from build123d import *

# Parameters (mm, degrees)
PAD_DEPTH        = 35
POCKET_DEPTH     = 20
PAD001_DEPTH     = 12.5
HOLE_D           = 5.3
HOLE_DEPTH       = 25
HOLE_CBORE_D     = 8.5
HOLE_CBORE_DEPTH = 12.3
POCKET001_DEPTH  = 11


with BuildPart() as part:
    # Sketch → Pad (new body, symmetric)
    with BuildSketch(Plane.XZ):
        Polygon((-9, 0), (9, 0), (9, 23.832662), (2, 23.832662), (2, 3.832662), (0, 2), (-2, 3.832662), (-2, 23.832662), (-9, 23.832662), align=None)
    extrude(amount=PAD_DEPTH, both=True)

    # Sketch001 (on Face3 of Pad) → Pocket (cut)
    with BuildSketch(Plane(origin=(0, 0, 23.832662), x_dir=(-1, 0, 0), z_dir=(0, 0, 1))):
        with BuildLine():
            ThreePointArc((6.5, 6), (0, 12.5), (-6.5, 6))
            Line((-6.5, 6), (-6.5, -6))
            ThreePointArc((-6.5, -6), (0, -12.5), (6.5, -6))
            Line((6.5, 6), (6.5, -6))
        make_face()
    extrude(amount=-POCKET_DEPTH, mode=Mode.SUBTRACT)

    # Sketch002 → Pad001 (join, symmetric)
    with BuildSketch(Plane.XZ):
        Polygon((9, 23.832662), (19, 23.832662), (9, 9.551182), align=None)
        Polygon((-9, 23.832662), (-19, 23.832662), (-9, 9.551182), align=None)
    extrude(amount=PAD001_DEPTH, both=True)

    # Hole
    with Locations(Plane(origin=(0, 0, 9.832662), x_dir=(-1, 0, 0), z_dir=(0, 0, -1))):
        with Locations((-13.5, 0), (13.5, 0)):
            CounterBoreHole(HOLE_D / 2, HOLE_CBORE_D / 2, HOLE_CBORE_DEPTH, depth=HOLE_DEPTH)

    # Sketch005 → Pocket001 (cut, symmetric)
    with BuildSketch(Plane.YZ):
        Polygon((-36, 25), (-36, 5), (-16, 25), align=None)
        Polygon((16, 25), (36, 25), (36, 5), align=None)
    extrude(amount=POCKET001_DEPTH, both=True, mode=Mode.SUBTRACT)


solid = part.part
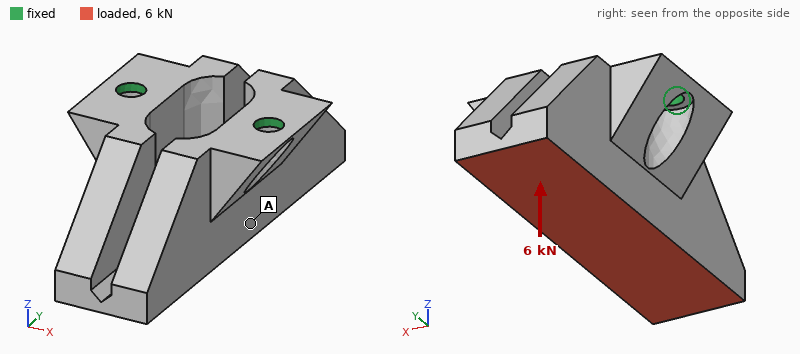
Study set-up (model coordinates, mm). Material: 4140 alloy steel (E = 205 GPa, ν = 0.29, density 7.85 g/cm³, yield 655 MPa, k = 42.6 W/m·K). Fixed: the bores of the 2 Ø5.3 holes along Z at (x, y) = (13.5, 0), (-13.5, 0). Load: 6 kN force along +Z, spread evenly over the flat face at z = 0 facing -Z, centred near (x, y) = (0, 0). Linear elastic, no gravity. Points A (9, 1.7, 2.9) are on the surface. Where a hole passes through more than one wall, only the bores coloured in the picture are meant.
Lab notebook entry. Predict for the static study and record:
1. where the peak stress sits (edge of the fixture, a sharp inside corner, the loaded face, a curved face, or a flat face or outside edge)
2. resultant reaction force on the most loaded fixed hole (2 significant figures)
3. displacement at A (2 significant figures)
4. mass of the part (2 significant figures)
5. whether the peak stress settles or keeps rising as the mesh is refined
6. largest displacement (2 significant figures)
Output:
edge of the fixture
3.2 kN
8.5 µm
150 g
keeps rising
16 µm
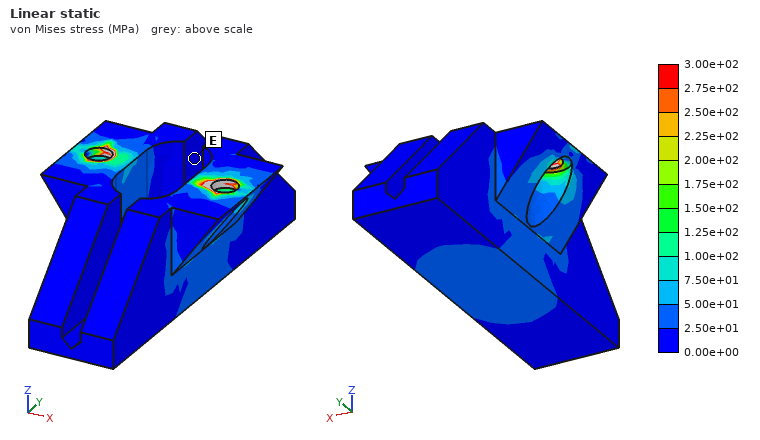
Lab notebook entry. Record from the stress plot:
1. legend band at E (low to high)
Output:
0.00e+00 to 2.50e+01 MPa
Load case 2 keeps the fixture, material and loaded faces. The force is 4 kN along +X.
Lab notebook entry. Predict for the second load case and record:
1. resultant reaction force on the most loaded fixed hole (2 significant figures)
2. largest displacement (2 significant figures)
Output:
4.0 kN
29 µm
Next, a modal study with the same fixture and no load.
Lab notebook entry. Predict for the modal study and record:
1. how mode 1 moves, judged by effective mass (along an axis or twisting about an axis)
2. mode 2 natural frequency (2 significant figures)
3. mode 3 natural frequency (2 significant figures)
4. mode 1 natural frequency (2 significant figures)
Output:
along Y
6900 Hz
7000 Hz
1500 Hz
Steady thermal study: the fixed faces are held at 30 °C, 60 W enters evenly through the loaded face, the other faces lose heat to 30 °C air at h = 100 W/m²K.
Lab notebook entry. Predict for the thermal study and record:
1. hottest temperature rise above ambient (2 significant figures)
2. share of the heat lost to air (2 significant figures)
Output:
71 K
62 %
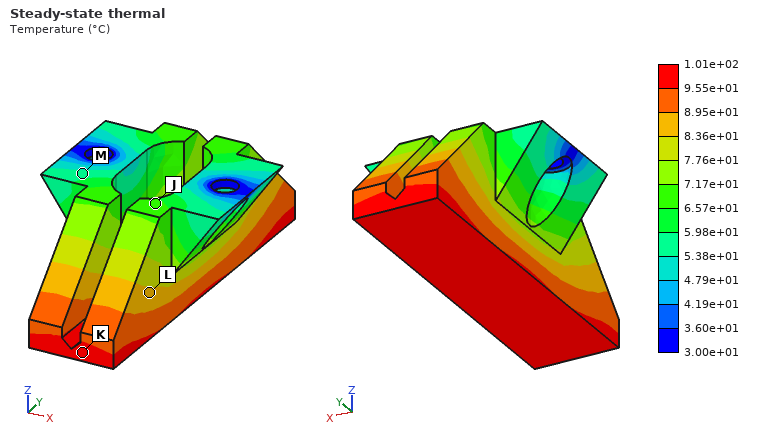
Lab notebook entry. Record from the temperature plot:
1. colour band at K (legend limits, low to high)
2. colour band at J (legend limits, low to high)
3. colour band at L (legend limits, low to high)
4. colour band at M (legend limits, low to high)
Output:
9.55e+01 to 1.01e+02 °C
6.57e+01 to 7.17e+01 °C
8.36e+01 to 8.95e+01 °C
5.38e+01 to 5.98e+01 °C
